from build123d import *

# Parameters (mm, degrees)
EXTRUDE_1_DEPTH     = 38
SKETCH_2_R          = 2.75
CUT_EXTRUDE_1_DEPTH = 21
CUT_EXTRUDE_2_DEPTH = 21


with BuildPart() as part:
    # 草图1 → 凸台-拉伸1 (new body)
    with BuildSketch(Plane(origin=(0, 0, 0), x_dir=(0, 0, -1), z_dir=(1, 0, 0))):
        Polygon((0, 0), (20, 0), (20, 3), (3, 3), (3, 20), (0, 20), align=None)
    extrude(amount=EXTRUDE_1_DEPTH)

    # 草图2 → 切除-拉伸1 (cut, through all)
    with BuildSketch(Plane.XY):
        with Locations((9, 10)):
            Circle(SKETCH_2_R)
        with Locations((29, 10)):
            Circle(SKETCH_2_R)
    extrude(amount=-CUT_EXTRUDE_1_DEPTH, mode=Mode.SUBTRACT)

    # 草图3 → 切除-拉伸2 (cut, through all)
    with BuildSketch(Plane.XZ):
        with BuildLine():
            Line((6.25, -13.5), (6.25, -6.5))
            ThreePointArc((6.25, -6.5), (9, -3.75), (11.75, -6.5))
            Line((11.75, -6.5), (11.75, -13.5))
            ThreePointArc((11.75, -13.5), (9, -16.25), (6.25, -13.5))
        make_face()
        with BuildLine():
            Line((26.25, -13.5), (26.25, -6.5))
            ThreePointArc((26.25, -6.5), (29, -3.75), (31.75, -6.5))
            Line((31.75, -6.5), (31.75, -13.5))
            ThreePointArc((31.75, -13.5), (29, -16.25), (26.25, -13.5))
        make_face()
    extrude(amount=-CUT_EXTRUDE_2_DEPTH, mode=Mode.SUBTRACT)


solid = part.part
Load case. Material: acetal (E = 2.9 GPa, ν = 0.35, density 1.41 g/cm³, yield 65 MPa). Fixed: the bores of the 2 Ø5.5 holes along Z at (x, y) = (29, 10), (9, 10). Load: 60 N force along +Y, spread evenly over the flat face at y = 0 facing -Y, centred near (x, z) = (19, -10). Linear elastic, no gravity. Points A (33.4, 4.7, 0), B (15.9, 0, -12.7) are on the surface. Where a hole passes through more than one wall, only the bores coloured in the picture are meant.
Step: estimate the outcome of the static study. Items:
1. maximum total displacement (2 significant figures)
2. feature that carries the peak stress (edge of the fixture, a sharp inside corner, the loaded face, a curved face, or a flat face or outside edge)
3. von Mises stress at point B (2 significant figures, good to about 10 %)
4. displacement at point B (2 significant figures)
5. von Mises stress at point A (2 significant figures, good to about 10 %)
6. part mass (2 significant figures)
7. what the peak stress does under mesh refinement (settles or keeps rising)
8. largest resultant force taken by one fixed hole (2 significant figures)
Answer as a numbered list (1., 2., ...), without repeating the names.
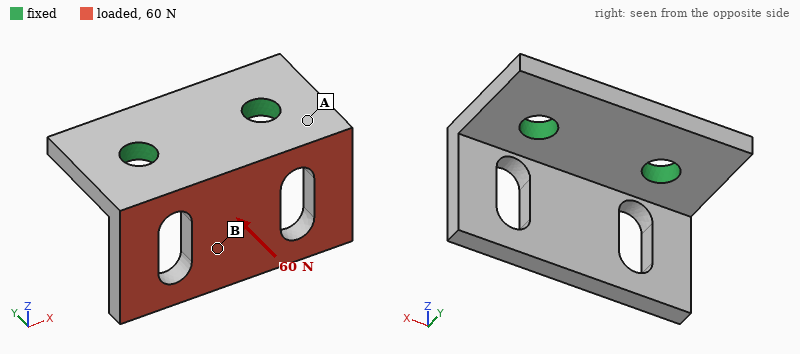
1. 0.46 mm
2. edge of the fixture
3. 2.2 MPa
4. 0.26 mm
5. 7.1 MPa
6. 5.2 g
7. keeps rising
8. 30 N
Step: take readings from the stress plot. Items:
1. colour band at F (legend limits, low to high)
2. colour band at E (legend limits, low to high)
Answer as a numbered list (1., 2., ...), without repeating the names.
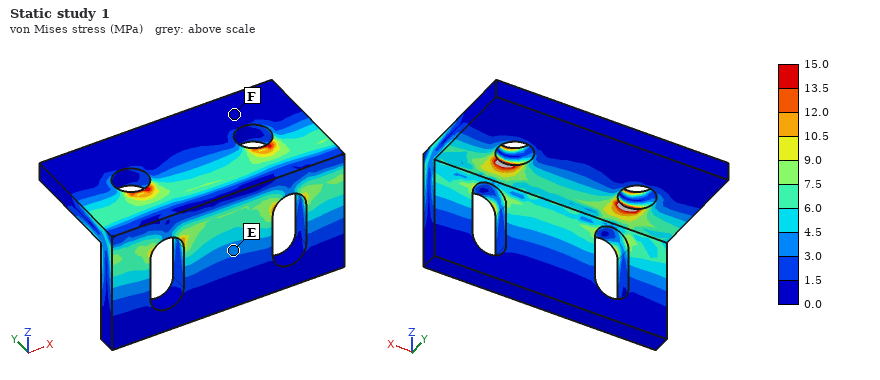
1. 0.0 to 1.5 MPa
2. 3.0 to 4.5 MPa
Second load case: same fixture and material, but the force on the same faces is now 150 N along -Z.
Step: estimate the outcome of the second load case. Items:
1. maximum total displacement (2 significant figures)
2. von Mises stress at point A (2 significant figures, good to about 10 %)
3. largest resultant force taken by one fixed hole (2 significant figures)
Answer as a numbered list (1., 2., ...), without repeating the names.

1. 0.52 mm
2. 10 MPa
3. 75 N
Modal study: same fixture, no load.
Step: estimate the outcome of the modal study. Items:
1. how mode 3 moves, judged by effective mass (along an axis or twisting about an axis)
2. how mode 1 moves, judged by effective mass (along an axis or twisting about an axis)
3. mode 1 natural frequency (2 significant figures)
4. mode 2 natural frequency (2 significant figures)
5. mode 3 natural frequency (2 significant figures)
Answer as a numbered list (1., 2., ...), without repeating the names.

1. along X
2. along Y
3. 1300 Hz
4. 2100 Hz
5. 3600 Hz
